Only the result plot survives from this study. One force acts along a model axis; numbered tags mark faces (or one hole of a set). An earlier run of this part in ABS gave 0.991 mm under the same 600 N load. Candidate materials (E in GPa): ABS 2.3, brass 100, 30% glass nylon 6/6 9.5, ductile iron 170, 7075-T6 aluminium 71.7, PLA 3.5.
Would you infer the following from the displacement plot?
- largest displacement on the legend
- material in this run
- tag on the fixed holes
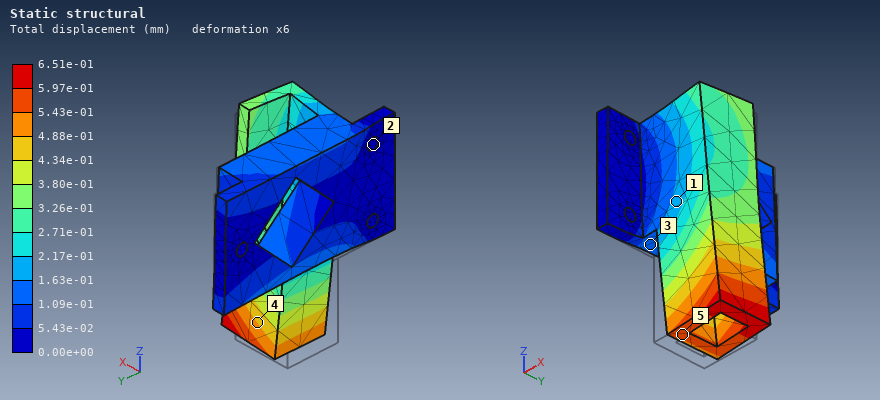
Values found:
6.51e-01 mm
PLA
2
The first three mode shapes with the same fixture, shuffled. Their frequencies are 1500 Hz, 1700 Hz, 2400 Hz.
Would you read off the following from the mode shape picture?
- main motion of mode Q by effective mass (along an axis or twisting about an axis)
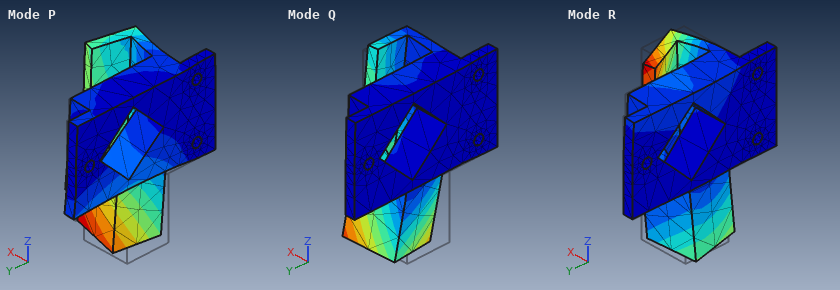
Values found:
along Y
